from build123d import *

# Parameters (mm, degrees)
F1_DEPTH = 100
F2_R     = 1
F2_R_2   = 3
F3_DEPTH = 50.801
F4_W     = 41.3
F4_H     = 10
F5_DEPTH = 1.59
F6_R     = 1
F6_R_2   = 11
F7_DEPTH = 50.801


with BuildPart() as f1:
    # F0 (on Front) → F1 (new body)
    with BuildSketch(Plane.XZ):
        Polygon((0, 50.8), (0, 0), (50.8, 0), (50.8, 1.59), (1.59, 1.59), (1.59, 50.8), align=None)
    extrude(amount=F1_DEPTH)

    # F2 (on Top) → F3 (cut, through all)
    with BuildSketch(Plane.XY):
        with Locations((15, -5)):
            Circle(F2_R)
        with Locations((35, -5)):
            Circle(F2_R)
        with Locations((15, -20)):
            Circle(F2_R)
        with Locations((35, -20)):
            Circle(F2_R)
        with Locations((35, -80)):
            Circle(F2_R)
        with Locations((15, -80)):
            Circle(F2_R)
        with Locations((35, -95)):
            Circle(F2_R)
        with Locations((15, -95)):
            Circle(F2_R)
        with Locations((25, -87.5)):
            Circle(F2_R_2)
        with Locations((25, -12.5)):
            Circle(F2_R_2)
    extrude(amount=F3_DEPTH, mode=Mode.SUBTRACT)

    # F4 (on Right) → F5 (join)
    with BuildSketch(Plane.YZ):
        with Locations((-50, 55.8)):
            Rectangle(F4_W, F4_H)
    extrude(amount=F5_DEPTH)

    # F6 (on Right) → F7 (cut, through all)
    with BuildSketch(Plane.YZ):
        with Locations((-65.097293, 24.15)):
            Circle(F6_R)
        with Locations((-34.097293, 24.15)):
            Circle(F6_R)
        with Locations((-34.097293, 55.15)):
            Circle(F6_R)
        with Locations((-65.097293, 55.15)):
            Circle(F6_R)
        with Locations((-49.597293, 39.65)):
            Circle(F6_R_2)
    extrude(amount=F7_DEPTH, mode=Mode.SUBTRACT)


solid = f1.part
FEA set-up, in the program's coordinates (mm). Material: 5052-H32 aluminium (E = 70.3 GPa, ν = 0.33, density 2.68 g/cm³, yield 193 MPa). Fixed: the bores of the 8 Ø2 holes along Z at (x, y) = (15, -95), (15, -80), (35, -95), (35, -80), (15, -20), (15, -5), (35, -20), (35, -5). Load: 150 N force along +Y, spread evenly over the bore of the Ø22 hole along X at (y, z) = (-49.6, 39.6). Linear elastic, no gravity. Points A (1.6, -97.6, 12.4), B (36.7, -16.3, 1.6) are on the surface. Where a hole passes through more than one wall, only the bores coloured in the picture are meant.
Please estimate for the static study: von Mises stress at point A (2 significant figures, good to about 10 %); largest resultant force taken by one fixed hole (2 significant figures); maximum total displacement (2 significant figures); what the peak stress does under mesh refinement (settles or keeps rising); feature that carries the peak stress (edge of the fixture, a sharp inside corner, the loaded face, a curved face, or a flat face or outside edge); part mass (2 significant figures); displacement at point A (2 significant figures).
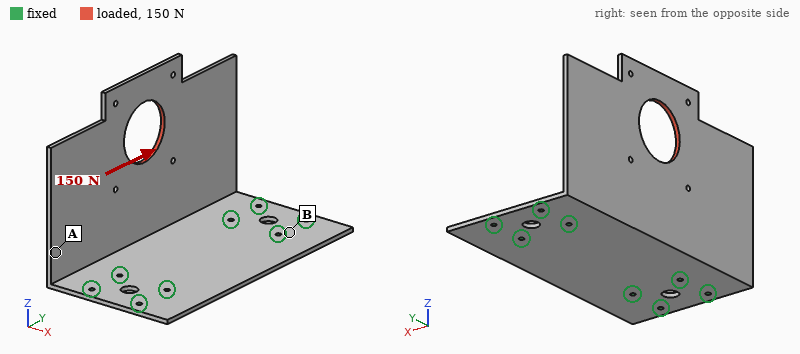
15 MPa
56 N
0.25 mm
keeps rising
edge of the fixture
42 g
0.12 mm
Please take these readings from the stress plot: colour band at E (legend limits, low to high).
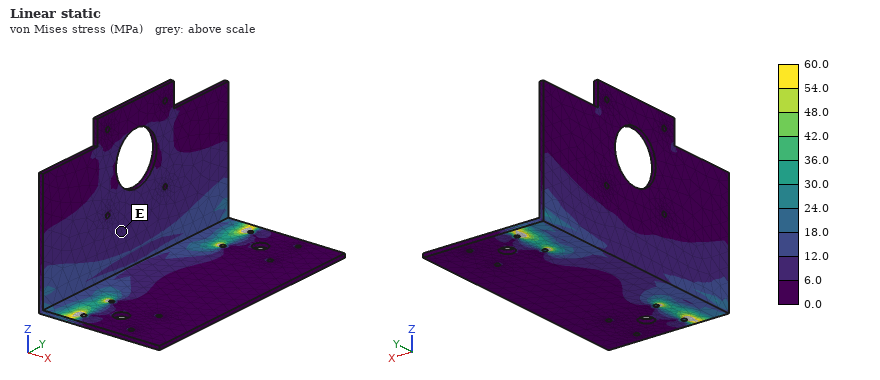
6.0 to 12.0 MPa
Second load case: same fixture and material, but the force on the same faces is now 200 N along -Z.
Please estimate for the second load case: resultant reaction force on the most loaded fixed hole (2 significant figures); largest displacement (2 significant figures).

84 N
0.61 mm
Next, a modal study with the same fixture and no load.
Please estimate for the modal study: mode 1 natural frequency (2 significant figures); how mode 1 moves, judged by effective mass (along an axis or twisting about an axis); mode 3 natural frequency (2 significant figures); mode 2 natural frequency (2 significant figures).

330 Hz
along X
1300 Hz
630 Hz
